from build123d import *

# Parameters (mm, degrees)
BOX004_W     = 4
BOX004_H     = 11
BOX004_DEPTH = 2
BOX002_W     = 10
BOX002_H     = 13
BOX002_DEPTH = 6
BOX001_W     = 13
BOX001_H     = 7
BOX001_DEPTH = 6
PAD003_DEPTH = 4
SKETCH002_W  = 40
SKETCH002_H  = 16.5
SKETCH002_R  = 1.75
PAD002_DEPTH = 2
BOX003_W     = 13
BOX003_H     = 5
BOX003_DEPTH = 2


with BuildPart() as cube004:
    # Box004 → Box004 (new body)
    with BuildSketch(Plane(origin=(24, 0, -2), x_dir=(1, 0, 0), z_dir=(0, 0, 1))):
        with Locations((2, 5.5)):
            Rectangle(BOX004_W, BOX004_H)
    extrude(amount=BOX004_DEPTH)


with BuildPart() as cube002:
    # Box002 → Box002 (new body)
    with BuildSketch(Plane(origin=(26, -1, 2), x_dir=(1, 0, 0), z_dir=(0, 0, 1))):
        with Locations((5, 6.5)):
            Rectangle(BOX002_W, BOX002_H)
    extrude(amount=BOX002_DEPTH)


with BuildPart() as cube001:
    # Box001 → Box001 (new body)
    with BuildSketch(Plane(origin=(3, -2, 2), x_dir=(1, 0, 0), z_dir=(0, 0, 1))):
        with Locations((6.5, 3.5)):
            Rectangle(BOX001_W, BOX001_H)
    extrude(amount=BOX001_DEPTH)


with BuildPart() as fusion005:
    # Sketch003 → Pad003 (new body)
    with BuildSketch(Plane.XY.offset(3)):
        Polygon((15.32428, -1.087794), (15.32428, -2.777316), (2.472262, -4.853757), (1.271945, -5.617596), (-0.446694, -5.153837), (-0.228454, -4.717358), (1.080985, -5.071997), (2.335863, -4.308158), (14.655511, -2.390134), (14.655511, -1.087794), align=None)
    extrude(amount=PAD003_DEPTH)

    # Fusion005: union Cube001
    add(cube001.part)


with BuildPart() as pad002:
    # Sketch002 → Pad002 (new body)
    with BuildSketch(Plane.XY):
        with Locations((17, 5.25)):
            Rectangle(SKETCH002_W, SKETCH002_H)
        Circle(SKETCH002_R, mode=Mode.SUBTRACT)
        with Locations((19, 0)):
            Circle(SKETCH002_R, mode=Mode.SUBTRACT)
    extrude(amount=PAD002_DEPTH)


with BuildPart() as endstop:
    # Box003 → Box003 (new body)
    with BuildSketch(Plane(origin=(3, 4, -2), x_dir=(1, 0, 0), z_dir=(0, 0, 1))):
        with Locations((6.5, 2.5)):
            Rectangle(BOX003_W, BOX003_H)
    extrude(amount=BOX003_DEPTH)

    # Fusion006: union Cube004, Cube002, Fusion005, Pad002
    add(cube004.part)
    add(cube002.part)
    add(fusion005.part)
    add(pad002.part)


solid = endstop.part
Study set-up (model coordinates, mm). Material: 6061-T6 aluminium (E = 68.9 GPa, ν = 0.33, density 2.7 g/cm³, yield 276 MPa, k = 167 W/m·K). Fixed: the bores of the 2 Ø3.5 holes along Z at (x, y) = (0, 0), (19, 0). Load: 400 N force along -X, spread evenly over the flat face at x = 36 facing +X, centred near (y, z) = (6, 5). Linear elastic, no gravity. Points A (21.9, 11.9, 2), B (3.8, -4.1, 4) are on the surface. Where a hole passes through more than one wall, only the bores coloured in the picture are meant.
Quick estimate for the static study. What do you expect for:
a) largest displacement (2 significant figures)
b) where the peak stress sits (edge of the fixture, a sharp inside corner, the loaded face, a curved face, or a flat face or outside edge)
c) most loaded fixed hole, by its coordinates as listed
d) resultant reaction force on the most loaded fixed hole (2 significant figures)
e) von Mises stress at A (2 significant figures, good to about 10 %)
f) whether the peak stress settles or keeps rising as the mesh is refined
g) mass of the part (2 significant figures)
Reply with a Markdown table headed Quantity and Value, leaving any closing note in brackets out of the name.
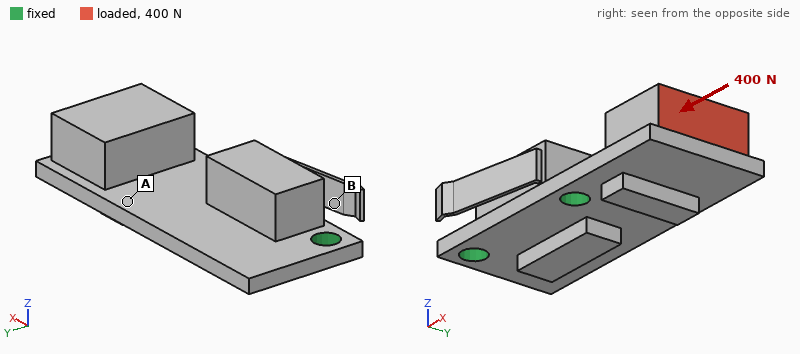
| Quantity | Value |
|---|---|
| largest displacement | 0.24 mm |
| where the peak stress sits | edge of the fixture |
| most loaded fixed hole, by its coordinates as listed | (19, 0) |
| resultant reaction force on the most loaded fixed hole | 300 N |
| von Mises stress at A | 110 MPa |
| whether the peak stress settles or keeps rising as the mesh is refined | keeps rising |
| mass of the part | 7.7 g |
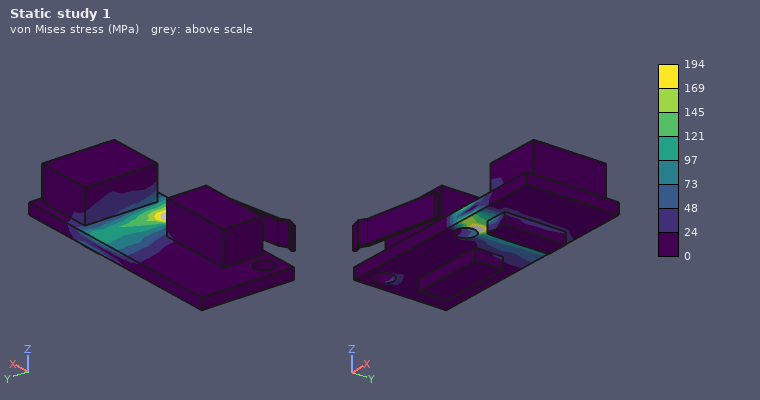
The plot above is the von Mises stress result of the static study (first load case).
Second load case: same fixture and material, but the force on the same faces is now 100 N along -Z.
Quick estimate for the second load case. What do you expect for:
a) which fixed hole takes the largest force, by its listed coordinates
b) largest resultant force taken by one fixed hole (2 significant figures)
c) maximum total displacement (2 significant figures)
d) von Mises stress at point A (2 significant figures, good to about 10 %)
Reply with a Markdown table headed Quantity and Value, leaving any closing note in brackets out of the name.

| Quantity | Value |
|---|---|
| which fixed hole takes the largest force, by its listed coordinates | (19, 0) |
| largest resultant force taken by one fixed hole | 130 N |
| maximum total displacement | 0.22 mm |
| von Mises stress at point A | 75 MPa |
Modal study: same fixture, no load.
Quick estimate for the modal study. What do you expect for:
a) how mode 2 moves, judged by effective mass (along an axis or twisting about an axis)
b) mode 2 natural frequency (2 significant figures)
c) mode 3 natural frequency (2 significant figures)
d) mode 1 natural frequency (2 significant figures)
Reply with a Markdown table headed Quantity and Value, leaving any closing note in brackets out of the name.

| Quantity | Value |
|---|---|
| how mode 2 moves, judged by effective mass | along Z |
| mode 2 natural frequency | 2800 Hz |
| mode 3 natural frequency | 7000 Hz |
| mode 1 natural frequency | 1600 Hz |
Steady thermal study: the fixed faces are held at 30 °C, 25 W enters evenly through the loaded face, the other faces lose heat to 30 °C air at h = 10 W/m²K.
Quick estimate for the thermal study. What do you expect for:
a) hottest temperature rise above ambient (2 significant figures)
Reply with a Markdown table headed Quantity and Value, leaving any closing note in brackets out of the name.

| Quantity | Value |
|---|---|
| hottest temperature rise above ambient | 58 K |
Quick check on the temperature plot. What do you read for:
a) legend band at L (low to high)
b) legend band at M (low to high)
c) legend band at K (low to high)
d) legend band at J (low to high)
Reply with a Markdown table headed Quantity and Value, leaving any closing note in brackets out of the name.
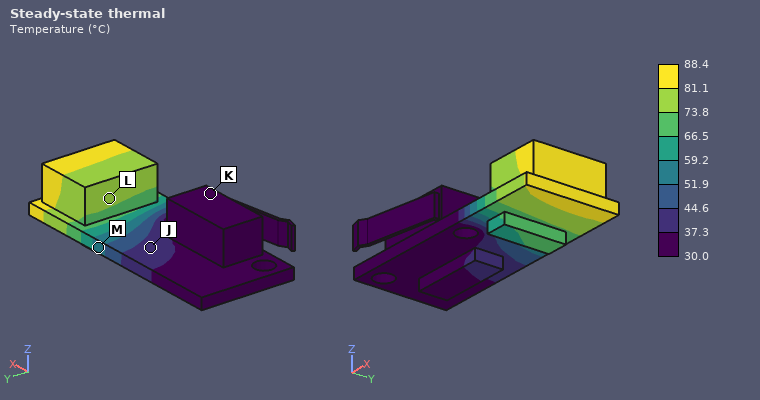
| Quantity | Value |
|---|---|
| legend band at L | 73.8 to 81.1 °C |
| legend band at M | 51.9 to 59.2 °C |
| legend band at K | 30.0 to 37.3 °C |
| legend band at J | 37.3 to 44.6 °C |
